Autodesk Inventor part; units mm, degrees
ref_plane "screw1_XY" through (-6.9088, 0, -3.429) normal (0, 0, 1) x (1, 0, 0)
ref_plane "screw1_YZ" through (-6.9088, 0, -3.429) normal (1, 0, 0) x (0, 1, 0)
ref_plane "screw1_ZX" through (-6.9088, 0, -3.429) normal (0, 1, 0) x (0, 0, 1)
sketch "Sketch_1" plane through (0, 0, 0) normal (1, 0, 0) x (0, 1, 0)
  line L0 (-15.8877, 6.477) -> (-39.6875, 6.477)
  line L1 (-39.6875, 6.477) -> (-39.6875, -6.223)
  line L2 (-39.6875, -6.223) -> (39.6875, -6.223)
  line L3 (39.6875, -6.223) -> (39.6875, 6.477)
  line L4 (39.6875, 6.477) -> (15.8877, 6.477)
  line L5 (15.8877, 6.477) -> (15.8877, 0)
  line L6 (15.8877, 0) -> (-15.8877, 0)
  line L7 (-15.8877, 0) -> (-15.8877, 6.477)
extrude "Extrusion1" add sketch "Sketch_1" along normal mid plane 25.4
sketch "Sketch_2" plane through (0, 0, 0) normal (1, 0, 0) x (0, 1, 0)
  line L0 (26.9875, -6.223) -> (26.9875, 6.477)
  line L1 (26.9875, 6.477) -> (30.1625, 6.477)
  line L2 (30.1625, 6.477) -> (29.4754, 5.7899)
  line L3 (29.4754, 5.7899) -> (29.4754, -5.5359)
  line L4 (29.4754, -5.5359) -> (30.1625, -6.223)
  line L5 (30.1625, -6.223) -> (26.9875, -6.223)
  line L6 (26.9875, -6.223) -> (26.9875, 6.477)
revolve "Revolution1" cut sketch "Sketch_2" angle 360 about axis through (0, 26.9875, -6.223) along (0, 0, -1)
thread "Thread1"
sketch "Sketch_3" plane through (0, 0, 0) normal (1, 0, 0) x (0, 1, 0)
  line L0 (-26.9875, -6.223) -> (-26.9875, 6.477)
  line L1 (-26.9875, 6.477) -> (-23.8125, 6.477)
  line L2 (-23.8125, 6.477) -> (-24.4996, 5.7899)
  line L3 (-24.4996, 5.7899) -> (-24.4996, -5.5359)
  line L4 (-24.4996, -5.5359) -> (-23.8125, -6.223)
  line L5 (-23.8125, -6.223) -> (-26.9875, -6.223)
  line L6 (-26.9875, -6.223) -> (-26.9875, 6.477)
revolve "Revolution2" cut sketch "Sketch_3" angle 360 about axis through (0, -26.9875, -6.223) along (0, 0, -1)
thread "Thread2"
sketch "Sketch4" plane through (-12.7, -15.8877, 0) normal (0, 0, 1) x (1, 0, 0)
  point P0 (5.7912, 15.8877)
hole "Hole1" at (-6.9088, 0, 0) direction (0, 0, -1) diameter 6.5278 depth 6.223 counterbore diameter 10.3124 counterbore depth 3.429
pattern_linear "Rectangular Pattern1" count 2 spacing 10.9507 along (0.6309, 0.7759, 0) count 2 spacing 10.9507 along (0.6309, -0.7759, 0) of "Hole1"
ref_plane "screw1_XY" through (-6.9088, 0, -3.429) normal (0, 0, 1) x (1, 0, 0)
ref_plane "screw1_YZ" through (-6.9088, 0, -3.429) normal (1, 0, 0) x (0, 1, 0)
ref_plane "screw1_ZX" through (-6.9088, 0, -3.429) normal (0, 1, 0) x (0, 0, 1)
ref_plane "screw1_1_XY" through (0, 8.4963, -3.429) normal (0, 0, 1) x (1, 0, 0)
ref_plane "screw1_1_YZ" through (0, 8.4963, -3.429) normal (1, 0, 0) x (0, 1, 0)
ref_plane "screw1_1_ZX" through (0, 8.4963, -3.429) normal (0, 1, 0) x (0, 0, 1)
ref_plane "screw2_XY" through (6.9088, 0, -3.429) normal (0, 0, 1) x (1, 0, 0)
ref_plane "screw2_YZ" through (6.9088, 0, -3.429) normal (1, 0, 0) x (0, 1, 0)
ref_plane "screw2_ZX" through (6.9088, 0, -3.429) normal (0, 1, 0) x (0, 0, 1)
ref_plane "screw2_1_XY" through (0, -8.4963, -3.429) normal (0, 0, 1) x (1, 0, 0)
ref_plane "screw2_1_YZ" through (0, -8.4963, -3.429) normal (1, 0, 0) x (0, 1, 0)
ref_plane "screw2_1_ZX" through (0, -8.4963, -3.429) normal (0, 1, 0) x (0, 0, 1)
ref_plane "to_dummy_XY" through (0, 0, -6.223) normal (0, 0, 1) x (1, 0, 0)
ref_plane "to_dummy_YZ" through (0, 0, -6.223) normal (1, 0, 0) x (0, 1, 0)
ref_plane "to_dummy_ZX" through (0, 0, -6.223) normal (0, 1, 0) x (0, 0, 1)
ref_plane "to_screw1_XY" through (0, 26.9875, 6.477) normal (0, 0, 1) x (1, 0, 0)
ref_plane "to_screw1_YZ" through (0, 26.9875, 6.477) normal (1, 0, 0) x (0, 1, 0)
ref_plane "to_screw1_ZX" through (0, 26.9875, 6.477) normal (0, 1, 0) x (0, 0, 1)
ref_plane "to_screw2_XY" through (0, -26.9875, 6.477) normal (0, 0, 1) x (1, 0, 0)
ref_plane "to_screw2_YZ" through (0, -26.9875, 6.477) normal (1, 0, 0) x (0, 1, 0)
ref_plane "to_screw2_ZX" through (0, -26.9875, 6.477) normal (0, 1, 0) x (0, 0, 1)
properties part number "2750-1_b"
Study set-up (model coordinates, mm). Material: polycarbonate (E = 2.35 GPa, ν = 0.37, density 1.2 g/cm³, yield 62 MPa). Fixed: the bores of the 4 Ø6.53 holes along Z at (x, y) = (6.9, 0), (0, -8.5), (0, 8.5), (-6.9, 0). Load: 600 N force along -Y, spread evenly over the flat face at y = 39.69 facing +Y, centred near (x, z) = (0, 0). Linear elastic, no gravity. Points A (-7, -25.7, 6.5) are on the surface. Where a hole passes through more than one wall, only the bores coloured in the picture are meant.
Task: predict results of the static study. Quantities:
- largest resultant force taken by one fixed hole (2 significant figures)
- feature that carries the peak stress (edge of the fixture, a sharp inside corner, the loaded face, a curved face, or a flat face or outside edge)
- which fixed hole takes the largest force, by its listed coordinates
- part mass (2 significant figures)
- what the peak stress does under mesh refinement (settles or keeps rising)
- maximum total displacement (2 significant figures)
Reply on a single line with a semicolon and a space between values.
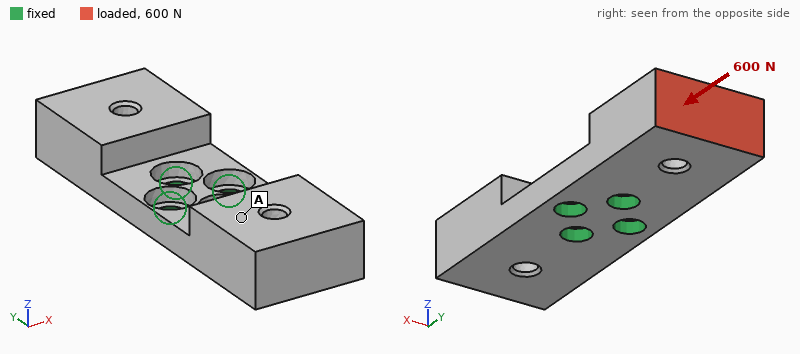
270 N; edge of the fixture; (0, 8.5); 22 g; keeps rising; 0.89 mm
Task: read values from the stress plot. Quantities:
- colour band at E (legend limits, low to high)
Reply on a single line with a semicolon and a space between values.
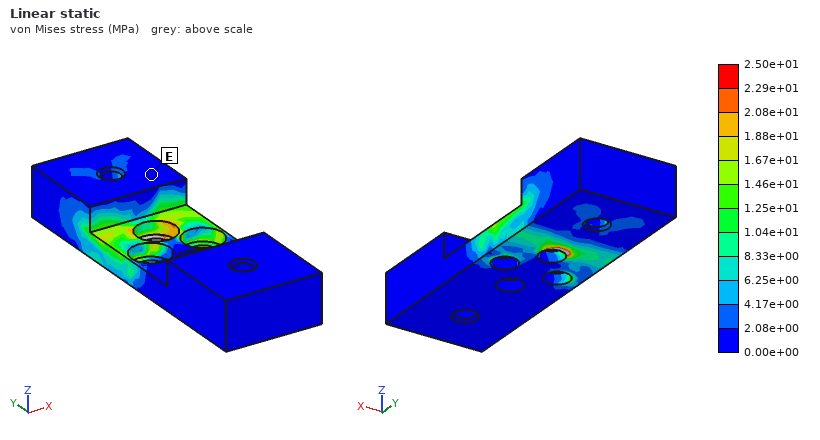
0.00e+00 to 2.08e+00 MPa
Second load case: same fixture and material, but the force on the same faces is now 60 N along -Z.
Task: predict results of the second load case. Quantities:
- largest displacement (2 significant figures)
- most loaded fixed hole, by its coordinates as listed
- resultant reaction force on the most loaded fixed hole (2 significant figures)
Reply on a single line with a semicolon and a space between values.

0.62 mm; (0, 8.5); 230 N
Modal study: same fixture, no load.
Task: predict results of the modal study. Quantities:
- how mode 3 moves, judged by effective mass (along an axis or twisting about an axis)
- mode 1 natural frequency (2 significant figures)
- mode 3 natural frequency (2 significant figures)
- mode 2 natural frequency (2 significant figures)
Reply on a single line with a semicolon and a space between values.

twisting about Z; 830 Hz; 2000 Hz; 830 Hz
